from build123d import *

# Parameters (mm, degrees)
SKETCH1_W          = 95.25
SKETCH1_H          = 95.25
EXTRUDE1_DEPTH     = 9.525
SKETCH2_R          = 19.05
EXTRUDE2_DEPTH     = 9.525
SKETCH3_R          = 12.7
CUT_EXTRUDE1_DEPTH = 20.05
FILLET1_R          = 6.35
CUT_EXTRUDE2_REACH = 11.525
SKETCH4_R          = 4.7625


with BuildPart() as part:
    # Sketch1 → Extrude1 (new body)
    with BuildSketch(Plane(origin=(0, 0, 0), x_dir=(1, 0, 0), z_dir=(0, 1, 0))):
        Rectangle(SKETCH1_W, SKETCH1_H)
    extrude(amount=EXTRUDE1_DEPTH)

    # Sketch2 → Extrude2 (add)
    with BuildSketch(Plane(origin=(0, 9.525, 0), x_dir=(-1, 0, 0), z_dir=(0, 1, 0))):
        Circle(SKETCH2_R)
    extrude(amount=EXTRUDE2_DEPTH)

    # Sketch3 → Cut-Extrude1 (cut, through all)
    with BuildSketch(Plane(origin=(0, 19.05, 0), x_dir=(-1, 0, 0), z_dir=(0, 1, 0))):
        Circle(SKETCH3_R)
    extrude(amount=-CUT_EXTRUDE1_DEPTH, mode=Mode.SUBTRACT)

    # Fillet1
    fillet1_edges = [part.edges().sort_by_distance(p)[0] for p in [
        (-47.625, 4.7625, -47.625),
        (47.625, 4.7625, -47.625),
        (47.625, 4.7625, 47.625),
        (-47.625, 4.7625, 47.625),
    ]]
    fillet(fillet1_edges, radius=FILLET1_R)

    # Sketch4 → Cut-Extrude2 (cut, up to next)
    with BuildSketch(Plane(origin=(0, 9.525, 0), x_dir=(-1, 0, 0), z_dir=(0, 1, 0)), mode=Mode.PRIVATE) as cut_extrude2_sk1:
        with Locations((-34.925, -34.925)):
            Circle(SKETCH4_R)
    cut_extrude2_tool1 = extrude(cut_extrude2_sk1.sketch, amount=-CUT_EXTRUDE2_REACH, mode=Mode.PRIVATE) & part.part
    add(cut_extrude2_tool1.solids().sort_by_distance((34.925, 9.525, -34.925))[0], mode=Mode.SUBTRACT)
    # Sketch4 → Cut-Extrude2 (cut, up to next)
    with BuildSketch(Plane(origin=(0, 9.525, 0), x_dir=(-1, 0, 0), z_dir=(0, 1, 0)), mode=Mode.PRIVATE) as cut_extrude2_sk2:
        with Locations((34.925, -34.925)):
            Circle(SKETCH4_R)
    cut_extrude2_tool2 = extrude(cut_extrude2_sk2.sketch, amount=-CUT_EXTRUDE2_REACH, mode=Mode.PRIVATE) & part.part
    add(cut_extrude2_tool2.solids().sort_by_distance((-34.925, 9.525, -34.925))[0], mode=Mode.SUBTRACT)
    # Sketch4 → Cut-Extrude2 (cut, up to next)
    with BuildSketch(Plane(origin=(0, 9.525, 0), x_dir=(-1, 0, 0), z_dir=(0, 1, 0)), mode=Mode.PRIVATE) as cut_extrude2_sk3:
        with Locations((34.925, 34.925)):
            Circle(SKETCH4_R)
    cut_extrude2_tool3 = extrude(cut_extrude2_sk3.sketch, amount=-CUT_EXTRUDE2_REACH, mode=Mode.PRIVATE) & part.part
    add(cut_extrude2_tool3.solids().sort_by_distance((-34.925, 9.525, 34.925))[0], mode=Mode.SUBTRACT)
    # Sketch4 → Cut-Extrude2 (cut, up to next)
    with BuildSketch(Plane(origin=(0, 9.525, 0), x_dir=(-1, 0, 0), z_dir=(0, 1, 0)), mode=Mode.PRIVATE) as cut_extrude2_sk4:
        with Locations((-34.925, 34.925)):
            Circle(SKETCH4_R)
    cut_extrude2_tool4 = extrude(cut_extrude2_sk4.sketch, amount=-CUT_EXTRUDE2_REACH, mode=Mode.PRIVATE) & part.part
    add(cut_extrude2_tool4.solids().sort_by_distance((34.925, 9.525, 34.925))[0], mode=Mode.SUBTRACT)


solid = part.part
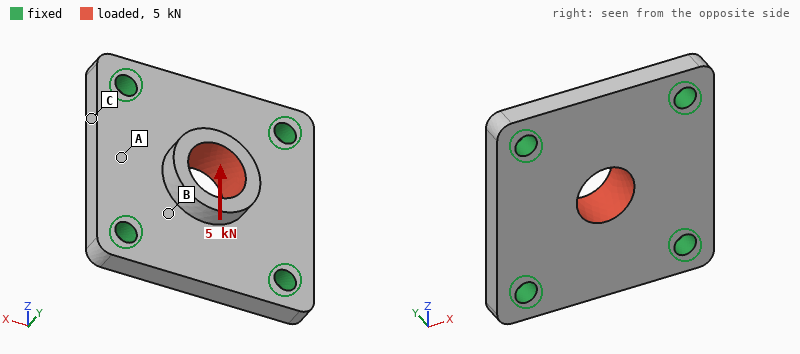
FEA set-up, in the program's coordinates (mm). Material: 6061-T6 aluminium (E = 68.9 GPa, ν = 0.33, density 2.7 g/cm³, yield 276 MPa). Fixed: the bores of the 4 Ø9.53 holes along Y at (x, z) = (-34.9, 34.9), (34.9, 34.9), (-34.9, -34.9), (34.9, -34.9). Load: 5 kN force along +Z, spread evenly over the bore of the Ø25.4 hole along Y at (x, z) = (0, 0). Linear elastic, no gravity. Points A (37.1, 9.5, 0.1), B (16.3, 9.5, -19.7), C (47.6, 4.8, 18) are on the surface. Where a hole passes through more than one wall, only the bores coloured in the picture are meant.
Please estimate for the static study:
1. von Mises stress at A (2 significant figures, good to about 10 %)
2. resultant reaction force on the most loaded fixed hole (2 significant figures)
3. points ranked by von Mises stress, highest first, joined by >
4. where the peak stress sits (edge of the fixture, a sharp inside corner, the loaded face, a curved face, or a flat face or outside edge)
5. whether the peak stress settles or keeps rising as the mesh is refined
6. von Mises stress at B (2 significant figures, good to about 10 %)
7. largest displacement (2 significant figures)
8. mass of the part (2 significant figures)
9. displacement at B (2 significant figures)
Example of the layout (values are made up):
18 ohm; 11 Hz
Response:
3.0 MPa; 1.4 kN; B > A > C; edge of the fixture; keeps rising; 8.5 MPa; 8.8 µm; 230 g; 3.3 µm
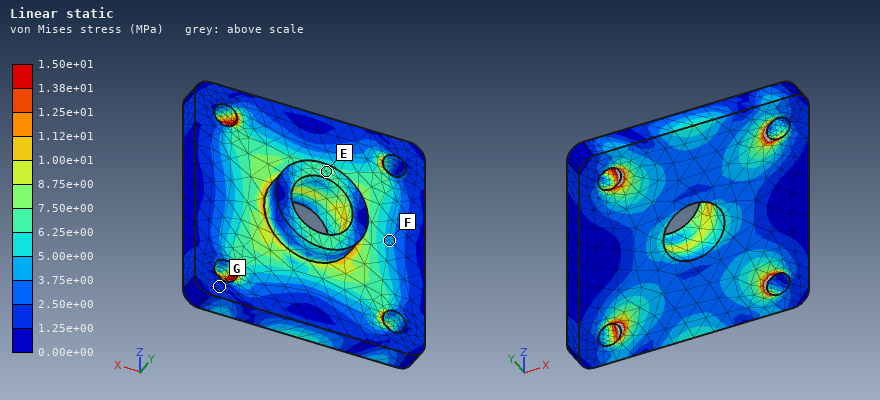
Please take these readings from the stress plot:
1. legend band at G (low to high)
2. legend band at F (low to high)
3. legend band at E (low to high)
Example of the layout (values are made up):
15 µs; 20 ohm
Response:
1.25e+00 to 2.50e+00 MPa; 3.75e+00 to 5.00e+00 MPa; 6.25e+00 to 7.50e+00 MPa
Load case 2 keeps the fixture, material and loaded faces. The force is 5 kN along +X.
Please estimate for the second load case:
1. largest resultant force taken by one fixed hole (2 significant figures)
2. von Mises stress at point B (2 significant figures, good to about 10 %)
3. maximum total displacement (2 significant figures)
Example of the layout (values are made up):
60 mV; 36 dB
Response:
1.4 kN; 8.6 MPa; 8.8 µm
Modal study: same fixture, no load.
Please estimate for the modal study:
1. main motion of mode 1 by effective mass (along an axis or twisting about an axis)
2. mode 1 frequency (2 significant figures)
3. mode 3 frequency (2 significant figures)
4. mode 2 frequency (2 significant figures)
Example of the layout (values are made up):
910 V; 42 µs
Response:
along Y; 7500 Hz; 11 kHz; 11 kHz
